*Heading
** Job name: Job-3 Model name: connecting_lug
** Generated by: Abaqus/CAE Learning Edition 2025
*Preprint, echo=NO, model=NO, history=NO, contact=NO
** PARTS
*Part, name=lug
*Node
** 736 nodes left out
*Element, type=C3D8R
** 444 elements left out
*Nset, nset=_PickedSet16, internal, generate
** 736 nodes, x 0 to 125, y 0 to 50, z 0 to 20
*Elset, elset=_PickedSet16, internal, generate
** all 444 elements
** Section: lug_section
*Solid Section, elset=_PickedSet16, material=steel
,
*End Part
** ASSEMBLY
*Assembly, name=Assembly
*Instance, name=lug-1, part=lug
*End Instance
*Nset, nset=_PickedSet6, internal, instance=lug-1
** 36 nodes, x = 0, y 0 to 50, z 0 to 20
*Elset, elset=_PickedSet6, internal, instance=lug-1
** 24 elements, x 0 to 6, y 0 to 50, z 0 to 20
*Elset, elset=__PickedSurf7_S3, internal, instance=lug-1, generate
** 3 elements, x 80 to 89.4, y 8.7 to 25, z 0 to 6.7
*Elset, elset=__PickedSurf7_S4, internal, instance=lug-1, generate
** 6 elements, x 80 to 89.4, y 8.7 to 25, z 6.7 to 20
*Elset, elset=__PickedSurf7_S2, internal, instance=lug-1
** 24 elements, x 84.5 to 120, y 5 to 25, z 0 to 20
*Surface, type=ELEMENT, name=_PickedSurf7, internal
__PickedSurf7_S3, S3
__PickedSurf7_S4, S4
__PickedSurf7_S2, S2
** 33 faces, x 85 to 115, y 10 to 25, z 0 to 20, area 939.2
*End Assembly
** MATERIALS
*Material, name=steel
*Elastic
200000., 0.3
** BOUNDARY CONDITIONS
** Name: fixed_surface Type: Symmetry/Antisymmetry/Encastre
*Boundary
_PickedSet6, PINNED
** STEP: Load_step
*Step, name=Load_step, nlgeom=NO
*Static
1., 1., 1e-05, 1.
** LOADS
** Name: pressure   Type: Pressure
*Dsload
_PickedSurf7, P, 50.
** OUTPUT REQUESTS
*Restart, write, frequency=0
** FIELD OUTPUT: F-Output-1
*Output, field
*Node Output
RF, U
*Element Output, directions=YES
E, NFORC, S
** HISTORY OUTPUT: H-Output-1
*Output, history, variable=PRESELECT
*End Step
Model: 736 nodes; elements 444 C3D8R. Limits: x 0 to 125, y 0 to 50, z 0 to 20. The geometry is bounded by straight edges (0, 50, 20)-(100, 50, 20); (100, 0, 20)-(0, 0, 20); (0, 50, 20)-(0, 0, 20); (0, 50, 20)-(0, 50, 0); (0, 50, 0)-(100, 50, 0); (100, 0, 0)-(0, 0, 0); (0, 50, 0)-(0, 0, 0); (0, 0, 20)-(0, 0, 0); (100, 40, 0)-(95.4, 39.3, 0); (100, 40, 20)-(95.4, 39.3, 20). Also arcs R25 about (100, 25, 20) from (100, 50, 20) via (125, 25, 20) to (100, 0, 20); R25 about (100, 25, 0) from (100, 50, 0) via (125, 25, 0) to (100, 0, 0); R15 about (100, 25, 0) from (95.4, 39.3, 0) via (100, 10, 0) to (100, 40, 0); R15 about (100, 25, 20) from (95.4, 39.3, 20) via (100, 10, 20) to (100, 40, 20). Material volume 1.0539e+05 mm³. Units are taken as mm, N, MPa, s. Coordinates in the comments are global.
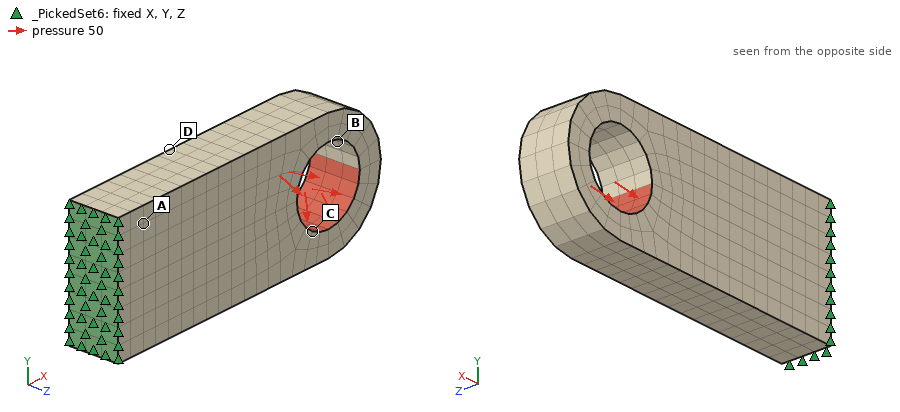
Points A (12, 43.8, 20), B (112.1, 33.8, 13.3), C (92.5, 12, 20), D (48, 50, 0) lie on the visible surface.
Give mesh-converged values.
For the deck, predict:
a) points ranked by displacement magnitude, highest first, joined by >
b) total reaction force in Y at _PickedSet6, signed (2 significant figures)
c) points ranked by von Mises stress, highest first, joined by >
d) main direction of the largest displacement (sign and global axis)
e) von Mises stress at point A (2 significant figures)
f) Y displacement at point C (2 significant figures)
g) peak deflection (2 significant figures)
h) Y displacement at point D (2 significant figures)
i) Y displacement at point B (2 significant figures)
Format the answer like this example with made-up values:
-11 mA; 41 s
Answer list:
B > C > D > A; 30000 N; C > B > A > D; -Y; 230 MPa; -0.26 mm; 0.42 mm; -0.091 mm; -0.38 mm
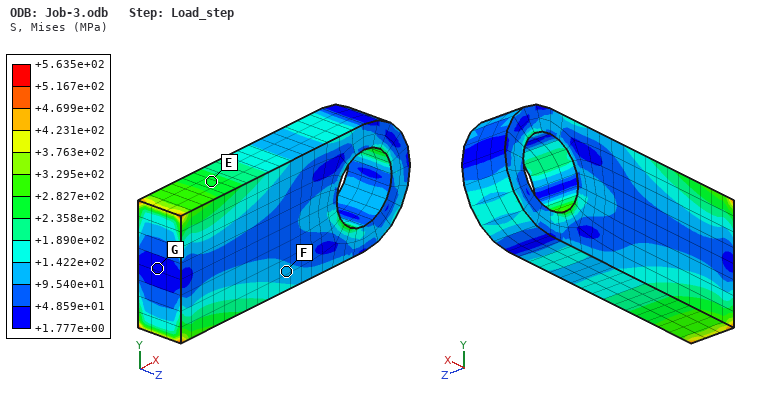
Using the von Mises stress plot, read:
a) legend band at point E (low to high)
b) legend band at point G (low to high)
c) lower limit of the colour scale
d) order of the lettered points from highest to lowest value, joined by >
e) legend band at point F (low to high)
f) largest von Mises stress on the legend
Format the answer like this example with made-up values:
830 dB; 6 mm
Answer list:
+2.358e+02 to +2.827e+02 MPa; +1.777e+00 to +4.859e+01 MPa; +1.777e+00 MPa; E > F > G; +9.540e+01 to +1.422e+02 MPa; +5.635e+02 MPa
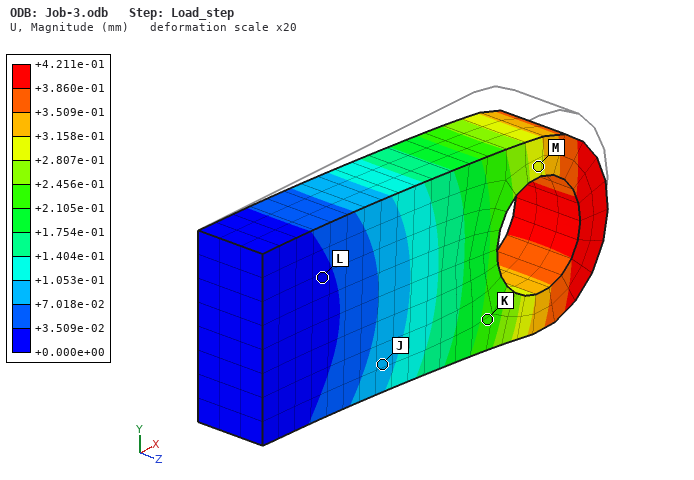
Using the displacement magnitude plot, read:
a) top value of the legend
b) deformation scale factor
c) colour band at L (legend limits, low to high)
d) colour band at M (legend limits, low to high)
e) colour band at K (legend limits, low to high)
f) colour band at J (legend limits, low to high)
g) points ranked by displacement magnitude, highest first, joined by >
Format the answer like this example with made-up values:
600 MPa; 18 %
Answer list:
+4.211e-01 mm; 20; +0.000e+00 to +3.509e-02 mm; +2.807e-01 to +3.158e-01 mm; +2.105e-01 to +2.456e-01 mm; +7.018e-02 to +1.053e-01 mm; M > K > J > L
